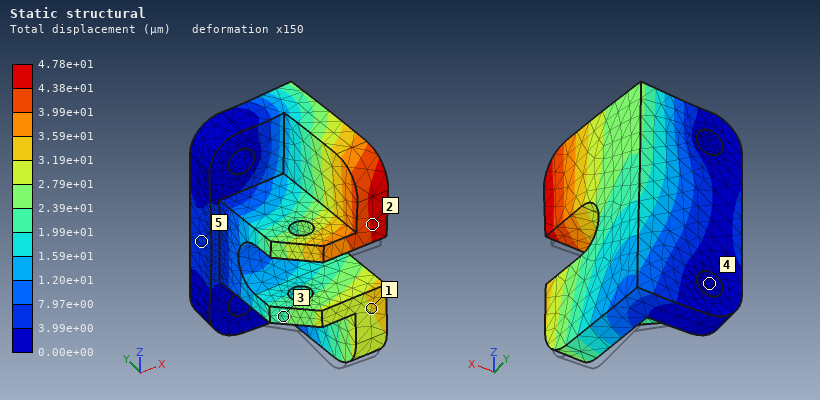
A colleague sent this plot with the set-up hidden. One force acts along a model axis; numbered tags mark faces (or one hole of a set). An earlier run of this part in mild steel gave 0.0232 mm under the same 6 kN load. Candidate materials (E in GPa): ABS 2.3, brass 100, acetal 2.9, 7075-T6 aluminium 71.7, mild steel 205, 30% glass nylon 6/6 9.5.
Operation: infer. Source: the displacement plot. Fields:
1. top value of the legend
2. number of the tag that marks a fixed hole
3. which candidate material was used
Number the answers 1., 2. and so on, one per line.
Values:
1. 4.78e+01 µm
2. 4
3. brass
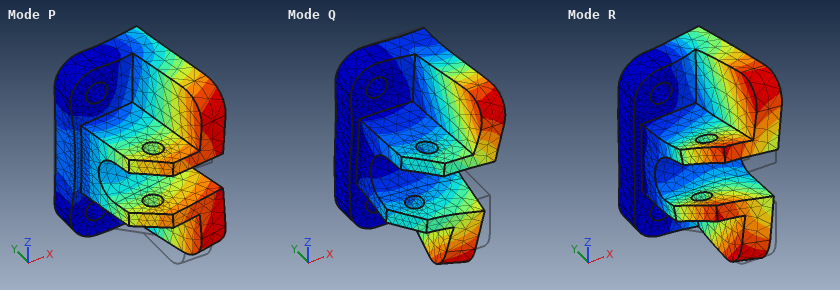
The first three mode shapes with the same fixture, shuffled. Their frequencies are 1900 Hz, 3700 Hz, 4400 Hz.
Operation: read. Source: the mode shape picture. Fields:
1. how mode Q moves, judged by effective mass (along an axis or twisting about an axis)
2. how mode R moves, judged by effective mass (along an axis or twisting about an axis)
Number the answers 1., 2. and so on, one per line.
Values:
1. along Z
2. along Z
